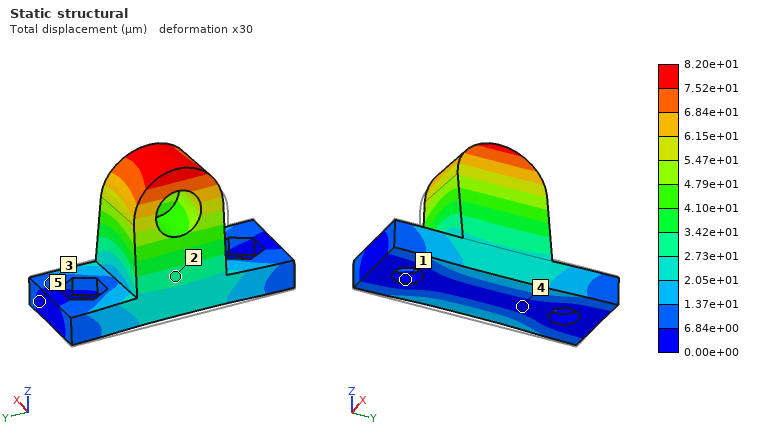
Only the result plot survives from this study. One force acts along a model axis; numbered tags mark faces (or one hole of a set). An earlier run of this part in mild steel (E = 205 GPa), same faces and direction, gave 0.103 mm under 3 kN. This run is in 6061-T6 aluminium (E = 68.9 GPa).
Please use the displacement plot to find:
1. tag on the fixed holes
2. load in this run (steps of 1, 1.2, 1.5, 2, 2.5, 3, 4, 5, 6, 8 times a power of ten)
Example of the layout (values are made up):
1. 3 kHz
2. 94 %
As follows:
1. 1
2. 800 N
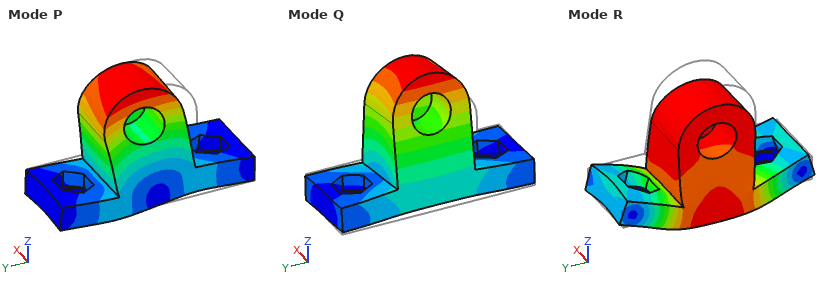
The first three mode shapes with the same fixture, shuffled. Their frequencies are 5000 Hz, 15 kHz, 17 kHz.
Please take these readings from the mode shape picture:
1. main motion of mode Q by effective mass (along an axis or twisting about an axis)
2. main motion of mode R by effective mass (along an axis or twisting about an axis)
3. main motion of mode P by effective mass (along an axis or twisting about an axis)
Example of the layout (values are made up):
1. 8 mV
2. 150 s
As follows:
1. along X
2. along Z
3. along Y
